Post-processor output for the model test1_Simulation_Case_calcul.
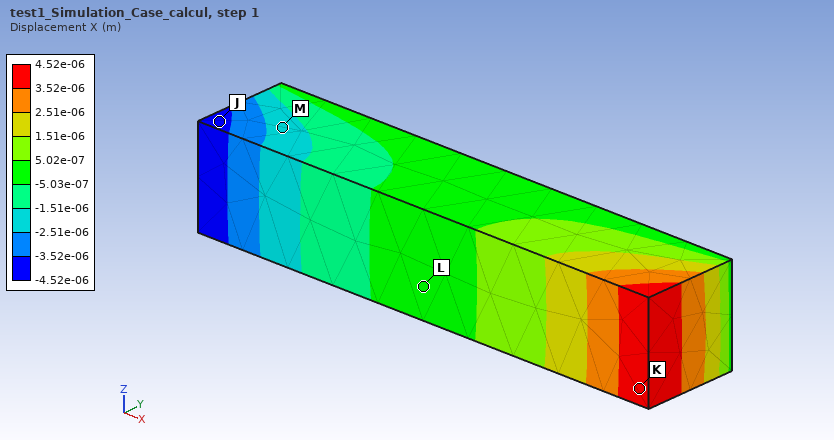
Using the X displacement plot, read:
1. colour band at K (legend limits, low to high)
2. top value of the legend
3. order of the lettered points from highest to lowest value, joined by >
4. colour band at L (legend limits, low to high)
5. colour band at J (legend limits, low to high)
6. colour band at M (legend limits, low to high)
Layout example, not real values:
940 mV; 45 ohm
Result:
3.52e-06 to 4.52e-06 m; 4.52e-06 m; K > L > M > J; -5.03e-07 to 5.02e-07 m; -4.52e-06 to -3.52e-06 m; -2.51e-06 to -1.51e-06 m
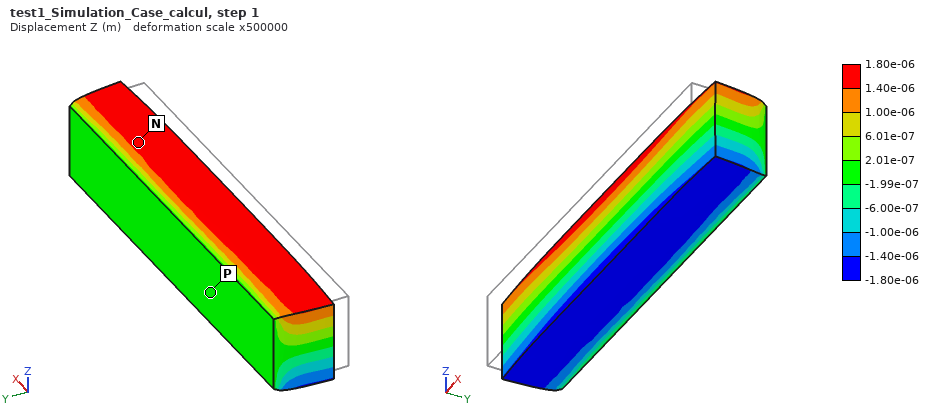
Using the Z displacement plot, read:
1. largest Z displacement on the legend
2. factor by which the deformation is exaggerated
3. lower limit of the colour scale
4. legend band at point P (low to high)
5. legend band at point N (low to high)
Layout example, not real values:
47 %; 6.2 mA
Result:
1.80e-06 m; 500000; -1.80e-06 m; -1.99e-07 to 2.01e-07 m; 1.40e-06 to 1.80e-06 m
